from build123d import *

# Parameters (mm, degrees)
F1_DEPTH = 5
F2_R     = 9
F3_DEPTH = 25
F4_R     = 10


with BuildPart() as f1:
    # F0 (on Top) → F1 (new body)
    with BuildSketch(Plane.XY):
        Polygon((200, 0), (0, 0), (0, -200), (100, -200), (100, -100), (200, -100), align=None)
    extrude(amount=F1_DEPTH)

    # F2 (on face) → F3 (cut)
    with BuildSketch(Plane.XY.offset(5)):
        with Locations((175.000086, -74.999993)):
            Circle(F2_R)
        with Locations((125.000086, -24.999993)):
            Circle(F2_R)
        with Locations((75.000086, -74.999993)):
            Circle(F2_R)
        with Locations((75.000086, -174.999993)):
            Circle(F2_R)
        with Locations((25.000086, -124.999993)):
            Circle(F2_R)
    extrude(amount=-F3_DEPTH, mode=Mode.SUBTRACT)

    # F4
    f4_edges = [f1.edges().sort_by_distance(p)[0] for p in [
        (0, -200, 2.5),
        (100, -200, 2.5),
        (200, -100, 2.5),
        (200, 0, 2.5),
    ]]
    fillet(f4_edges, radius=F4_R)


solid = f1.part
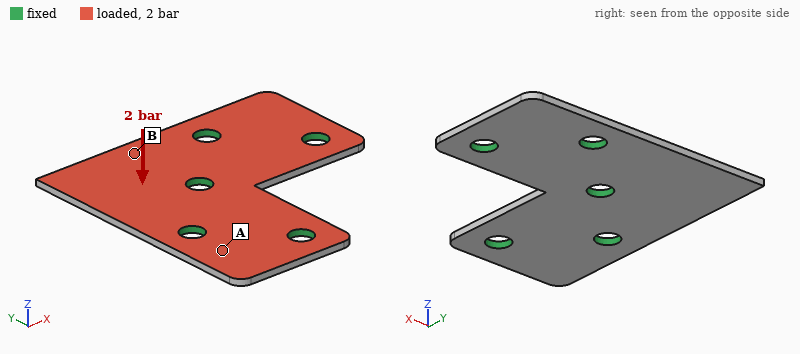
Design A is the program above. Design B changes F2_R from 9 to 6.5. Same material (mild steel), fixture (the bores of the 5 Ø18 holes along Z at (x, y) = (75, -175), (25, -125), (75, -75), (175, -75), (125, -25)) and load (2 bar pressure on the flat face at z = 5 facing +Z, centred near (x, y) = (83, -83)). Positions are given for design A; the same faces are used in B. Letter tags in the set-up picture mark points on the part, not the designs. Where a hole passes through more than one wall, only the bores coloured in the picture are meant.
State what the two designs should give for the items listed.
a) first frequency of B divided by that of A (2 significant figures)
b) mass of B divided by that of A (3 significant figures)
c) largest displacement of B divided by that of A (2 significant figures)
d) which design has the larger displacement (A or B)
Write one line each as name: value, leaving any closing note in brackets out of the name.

first frequency of B divided by that of A: 0.94
mass of B divided by that of A: 1.02
largest displacement of B divided by that of A: 1.1
which design has the larger displacement: B
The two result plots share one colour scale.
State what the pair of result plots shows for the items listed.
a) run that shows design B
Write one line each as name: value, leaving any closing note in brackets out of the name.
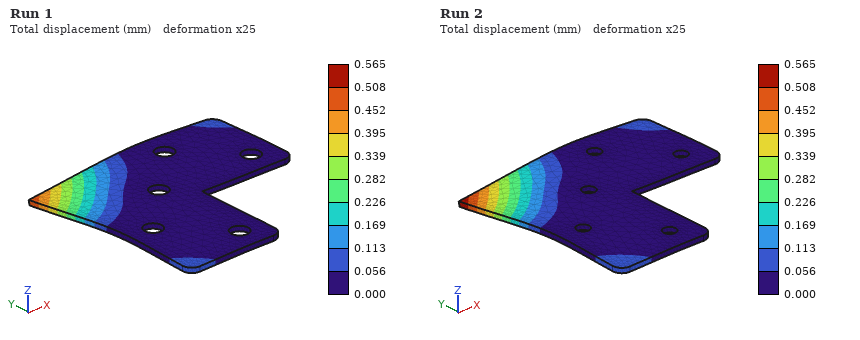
run that shows design B: Run 2
